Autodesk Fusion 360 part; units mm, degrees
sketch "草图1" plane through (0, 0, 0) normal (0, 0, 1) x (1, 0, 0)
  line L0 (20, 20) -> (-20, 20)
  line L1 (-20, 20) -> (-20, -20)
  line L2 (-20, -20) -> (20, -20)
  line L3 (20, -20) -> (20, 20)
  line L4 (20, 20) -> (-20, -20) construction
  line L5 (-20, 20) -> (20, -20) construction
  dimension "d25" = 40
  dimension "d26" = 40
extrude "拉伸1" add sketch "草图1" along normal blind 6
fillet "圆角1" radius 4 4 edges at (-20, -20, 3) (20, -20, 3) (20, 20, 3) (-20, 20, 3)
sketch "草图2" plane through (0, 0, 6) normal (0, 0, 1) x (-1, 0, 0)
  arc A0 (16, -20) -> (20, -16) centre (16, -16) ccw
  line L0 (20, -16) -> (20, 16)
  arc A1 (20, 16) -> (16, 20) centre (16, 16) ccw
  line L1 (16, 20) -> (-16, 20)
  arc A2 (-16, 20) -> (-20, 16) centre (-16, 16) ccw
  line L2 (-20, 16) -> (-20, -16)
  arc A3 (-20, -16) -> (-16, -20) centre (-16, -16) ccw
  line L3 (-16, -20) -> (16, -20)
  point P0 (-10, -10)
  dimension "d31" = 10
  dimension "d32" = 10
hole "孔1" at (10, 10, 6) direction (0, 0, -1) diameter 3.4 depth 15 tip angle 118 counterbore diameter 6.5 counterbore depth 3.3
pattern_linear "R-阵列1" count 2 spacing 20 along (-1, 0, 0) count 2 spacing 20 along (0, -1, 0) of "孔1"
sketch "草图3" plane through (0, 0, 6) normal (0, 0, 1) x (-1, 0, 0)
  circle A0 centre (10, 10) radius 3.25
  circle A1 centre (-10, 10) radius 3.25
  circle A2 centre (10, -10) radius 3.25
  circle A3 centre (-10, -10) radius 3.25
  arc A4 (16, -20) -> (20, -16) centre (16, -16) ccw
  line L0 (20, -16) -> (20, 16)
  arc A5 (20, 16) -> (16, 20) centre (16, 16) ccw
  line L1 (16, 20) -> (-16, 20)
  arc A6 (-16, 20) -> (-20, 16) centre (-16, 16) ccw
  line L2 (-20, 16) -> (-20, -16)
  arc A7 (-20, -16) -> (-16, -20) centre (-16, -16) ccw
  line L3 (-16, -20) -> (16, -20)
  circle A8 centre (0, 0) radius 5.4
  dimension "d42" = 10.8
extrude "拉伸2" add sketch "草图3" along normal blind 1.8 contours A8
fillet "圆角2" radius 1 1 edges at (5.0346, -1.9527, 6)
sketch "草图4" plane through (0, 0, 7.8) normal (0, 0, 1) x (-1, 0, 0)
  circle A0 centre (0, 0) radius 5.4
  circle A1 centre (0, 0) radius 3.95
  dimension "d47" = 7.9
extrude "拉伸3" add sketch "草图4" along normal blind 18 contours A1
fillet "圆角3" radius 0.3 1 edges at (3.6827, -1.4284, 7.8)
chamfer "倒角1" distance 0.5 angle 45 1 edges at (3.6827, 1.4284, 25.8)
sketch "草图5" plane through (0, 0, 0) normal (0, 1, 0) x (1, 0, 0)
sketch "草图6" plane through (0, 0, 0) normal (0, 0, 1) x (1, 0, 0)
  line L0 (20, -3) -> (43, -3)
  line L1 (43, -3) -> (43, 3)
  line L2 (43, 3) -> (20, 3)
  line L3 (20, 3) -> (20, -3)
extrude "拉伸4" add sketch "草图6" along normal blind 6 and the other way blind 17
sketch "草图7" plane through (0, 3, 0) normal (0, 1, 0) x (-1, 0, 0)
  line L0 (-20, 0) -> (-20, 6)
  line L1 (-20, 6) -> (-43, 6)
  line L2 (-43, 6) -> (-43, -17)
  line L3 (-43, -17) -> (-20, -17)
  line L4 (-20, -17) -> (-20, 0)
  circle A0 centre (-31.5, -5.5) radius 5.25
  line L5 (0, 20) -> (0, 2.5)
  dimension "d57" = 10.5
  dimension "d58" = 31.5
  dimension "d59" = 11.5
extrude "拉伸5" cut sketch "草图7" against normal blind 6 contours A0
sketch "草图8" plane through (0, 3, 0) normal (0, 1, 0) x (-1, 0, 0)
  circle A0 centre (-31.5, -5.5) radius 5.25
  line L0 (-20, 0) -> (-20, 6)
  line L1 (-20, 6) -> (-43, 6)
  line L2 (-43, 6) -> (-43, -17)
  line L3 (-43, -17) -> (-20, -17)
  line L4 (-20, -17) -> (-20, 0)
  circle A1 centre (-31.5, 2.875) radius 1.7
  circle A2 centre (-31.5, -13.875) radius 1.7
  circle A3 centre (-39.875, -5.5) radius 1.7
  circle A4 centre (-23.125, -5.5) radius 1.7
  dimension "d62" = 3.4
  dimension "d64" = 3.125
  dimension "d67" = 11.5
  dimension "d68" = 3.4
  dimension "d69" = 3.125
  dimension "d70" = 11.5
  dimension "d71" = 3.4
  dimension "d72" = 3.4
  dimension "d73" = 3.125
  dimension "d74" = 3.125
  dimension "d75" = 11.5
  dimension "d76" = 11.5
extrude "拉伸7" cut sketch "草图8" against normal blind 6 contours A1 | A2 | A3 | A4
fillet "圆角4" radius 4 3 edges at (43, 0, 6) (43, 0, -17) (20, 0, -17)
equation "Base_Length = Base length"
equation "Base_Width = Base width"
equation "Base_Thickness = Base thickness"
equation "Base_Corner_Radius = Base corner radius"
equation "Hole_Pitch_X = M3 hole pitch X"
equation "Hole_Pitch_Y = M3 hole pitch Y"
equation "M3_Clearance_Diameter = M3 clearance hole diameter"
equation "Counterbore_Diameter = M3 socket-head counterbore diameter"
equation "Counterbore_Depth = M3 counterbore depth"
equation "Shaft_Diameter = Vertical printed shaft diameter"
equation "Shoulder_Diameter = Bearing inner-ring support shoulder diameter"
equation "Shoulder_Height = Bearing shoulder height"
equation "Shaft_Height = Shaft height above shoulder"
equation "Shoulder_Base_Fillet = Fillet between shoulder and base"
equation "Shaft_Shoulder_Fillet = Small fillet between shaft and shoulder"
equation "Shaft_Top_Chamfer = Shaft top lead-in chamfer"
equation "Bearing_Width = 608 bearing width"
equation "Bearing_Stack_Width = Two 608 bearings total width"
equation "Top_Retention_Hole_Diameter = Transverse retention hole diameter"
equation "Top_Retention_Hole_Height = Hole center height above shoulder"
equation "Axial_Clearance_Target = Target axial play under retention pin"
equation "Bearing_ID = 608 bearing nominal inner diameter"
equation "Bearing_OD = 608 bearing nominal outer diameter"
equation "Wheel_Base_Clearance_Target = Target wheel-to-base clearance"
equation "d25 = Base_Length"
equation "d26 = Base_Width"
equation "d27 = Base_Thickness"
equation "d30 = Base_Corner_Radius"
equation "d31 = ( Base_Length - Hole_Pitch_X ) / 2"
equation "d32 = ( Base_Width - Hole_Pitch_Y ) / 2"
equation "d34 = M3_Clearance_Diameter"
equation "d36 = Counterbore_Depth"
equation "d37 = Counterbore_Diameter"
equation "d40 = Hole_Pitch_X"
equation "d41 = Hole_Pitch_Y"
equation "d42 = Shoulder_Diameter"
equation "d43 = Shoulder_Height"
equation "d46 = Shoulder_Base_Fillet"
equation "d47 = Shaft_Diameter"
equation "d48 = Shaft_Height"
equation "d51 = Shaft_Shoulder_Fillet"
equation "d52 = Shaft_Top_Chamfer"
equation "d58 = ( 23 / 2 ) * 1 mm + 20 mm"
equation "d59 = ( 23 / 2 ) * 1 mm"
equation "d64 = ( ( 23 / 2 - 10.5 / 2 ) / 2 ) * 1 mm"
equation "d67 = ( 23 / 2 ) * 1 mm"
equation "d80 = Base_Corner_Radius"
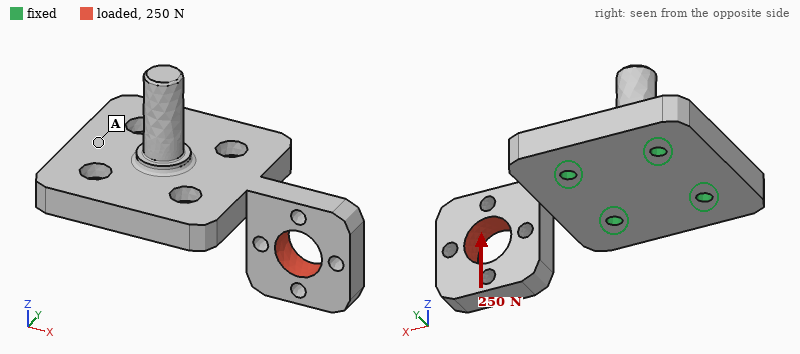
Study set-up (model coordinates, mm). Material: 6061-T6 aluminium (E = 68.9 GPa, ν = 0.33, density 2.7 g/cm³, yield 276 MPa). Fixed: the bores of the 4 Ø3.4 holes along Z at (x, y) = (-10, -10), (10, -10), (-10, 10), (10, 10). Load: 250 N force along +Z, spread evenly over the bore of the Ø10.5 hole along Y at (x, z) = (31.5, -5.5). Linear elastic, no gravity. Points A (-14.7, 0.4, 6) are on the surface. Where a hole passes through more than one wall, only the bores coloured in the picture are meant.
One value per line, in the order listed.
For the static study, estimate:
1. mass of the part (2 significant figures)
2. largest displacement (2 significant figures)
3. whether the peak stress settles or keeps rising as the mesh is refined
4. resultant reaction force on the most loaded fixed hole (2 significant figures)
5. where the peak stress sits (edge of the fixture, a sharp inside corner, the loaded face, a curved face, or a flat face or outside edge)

34 g
0.14 mm
keeps rising
320 N
edge of the fixture
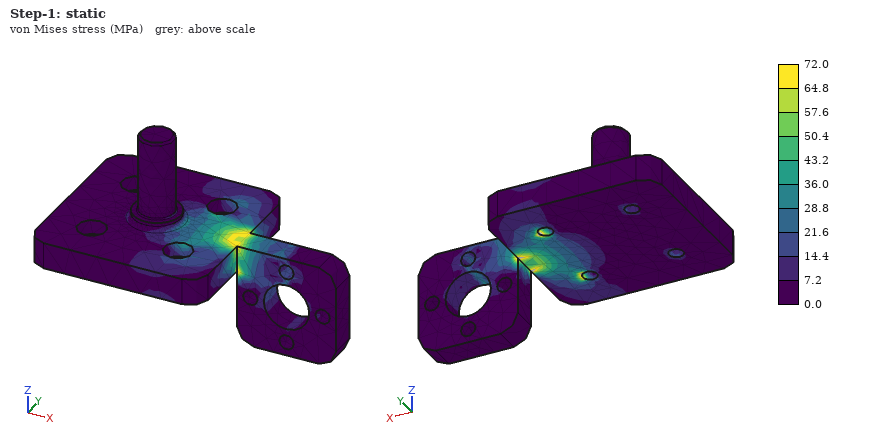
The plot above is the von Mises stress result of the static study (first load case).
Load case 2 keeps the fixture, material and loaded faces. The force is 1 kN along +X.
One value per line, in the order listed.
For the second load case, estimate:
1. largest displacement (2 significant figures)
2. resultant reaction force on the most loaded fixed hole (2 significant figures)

0.32 mm
690 N
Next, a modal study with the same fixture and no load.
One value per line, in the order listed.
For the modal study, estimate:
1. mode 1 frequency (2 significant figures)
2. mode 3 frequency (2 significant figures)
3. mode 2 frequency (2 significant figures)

2900 Hz
7400 Hz
3700 Hz
